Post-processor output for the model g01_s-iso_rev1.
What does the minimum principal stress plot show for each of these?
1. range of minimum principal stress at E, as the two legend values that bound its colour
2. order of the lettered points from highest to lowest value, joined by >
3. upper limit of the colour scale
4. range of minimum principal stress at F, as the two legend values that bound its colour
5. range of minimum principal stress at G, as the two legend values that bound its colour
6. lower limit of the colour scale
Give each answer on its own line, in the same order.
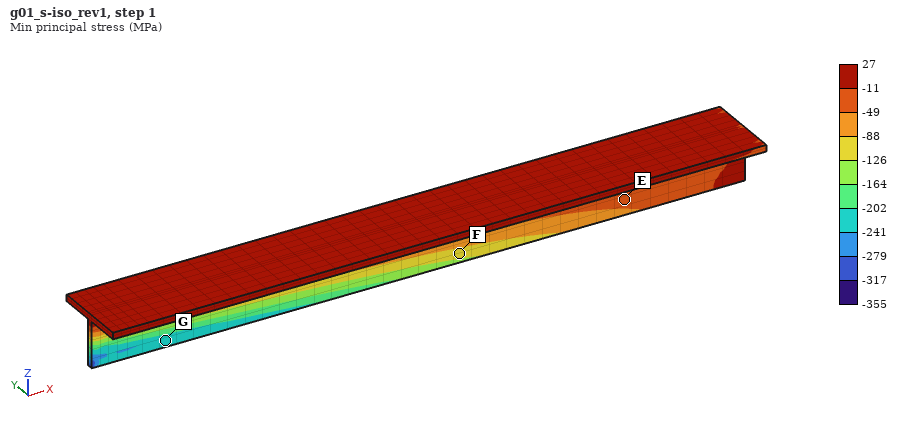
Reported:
-49 to -11 MPa
E > F > G
27 MPa
-126 to -88 MPa
-241 to -202 MPa
-355 MPa
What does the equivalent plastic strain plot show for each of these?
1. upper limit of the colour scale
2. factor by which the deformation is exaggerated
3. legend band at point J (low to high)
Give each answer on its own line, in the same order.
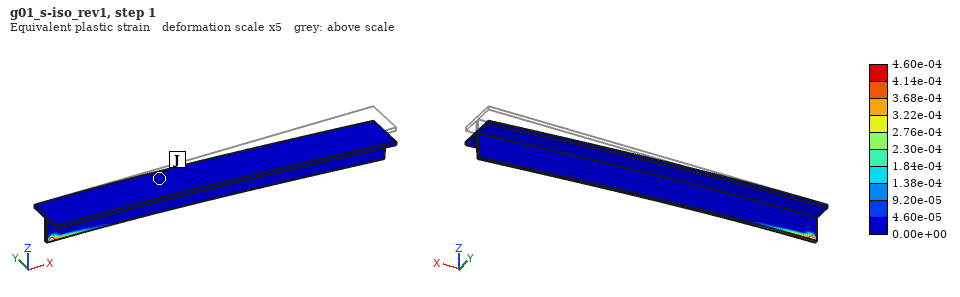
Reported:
4.60e-04
5
0.00e+00 to 4.60e-05
